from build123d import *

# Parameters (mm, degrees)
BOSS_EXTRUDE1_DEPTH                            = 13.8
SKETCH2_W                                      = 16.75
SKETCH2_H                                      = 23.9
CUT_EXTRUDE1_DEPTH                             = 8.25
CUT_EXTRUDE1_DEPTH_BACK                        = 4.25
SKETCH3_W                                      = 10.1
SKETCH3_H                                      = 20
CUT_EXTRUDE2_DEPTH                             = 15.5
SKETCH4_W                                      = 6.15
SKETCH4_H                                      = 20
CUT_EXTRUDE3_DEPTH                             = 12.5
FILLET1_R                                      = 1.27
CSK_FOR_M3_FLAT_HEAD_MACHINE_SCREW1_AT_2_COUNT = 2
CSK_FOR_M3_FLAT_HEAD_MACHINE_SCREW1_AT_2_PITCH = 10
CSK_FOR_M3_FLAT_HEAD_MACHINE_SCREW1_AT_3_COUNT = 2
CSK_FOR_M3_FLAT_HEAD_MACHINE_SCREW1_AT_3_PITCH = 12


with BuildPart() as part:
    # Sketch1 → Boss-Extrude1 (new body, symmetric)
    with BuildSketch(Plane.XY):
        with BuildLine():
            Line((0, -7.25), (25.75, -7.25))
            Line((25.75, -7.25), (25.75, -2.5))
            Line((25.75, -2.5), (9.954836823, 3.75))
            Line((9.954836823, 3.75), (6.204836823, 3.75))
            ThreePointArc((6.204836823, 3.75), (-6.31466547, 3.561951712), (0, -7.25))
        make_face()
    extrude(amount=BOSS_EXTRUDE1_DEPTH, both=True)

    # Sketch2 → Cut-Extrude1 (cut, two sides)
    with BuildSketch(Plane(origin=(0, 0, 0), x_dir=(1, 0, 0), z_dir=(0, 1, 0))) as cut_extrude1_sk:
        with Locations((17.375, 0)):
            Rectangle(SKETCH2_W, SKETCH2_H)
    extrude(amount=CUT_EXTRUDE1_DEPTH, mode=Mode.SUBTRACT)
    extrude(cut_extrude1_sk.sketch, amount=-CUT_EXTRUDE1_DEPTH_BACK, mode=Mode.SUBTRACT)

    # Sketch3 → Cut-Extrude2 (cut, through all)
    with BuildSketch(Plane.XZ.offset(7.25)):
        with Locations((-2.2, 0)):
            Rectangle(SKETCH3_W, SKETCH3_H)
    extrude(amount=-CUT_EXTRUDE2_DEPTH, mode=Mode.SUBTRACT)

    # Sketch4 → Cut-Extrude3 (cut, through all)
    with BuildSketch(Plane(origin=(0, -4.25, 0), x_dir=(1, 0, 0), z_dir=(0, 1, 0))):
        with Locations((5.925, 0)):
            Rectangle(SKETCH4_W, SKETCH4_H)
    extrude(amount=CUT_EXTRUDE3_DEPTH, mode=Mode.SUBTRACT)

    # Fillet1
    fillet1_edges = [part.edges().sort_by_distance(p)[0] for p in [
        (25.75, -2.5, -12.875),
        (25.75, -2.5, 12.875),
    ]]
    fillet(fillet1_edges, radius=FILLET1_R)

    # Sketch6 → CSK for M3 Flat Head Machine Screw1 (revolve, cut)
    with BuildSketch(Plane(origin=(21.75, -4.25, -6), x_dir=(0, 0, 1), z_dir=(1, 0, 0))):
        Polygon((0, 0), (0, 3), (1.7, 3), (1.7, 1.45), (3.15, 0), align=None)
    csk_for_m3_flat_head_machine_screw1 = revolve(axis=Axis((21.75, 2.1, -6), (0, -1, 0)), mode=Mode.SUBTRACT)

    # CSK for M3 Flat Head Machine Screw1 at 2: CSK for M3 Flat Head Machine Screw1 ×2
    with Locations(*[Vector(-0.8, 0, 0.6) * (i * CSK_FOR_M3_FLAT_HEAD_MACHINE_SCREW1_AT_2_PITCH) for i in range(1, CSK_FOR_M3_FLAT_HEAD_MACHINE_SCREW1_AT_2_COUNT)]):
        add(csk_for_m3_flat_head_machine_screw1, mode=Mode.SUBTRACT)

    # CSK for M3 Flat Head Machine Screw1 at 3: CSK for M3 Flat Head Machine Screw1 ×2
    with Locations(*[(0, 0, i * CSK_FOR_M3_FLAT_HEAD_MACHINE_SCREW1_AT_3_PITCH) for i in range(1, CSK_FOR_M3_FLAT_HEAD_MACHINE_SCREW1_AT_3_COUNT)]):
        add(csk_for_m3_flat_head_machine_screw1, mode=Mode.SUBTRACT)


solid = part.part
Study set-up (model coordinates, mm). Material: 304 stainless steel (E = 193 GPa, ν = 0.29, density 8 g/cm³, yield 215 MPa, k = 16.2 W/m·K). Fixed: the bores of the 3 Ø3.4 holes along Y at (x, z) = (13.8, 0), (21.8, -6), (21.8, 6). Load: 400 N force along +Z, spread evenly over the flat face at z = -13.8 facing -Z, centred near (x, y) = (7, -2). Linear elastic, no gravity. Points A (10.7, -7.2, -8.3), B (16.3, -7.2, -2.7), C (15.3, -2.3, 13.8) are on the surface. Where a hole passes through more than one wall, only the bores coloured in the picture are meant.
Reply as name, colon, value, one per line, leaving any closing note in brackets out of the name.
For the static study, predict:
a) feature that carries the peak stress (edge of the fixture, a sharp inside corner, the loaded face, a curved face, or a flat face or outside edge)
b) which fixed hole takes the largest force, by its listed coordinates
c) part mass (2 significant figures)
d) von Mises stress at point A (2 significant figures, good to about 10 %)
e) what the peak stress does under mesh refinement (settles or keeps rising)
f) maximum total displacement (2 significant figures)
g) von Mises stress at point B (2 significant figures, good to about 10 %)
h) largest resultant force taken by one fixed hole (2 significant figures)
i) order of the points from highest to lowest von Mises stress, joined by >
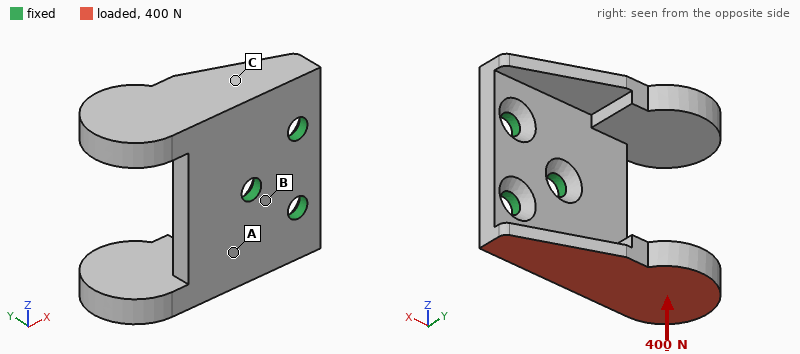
feature that carries the peak stress: edge of the fixture
which fixed hole takes the largest force, by its listed coordinates: (13.8, 0)
part mass: 28 g
von Mises stress at point A: 49 MPa
what the peak stress does under mesh refinement: keeps rising
maximum total displacement: 54 µm
von Mises stress at point B: 30 MPa
largest resultant force taken by one fixed hole: 390 N
order of the points from highest to lowest von Mises stress, joined by >: A > B > C
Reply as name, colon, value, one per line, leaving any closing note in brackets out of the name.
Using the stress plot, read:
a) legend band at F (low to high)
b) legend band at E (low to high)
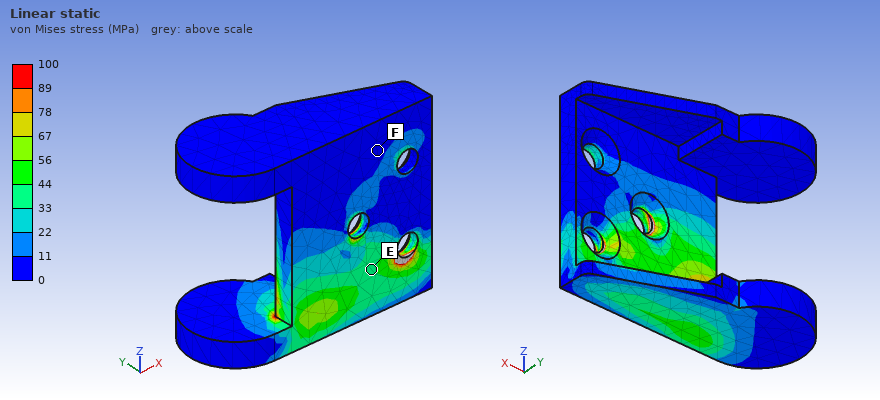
legend band at F: 0 to 11 MPa
legend band at E: 33 to 44 MPa
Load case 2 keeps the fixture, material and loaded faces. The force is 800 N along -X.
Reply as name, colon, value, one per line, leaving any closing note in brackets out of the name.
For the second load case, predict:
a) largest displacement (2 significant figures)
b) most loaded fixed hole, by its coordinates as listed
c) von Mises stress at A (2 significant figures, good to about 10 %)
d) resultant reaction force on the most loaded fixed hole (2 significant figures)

largest displacement: 60 µm
most loaded fixed hole, by its coordinates as listed: (21.8, -6)
von Mises stress at A: 29 MPa
resultant reaction force on the most loaded fixed hole: 880 N
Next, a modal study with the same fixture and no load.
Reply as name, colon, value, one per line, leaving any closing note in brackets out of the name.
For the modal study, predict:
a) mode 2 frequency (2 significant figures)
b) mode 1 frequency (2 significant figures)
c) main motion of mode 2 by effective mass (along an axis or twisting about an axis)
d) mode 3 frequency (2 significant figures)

mode 2 frequency: 3800 Hz
mode 1 frequency: 3400 Hz
main motion of mode 2 by effective mass: along Y
mode 3 frequency: 8100 Hz
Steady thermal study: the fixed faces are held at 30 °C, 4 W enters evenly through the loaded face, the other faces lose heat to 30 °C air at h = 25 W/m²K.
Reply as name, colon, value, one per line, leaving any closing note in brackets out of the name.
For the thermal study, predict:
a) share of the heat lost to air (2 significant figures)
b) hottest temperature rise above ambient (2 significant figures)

share of the heat lost to air: 23 %
hottest temperature rise above ambient: 61 K
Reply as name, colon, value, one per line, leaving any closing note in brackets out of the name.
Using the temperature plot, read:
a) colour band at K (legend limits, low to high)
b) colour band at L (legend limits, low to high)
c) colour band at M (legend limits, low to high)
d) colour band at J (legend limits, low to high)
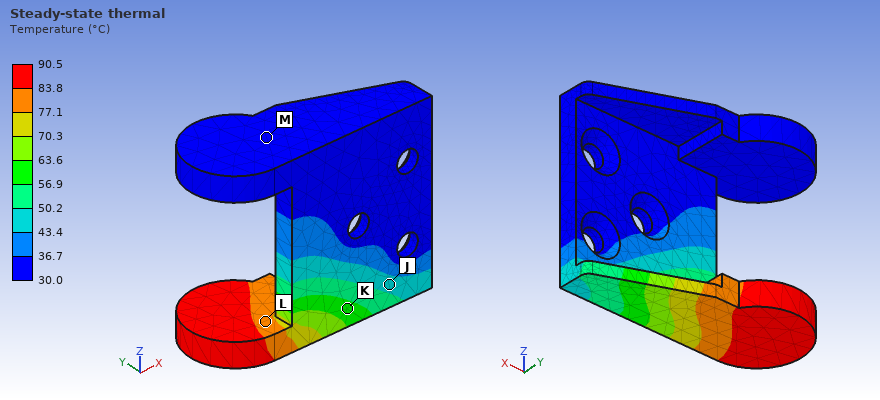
colour band at K: 56.9 to 63.6 °C
colour band at L: 77.1 to 83.8 °C
colour band at M: 30.0 to 36.7 °C
colour band at J: 43.4 to 50.2 °C
